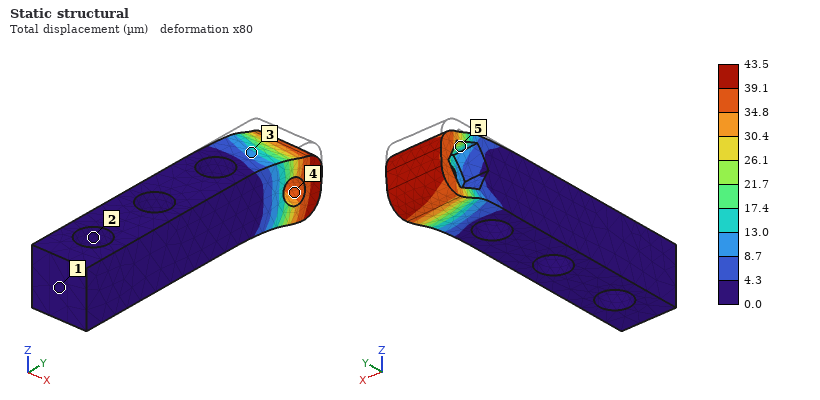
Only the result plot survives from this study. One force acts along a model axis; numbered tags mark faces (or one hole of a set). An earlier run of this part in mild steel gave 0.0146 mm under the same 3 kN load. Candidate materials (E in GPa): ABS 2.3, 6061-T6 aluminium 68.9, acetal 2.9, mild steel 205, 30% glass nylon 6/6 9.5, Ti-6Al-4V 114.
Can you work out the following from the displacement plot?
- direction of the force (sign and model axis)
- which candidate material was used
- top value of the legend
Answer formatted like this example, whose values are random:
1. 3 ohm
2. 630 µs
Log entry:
1. -Z
2. 6061-T6 aluminium
3. 43.5 µm
